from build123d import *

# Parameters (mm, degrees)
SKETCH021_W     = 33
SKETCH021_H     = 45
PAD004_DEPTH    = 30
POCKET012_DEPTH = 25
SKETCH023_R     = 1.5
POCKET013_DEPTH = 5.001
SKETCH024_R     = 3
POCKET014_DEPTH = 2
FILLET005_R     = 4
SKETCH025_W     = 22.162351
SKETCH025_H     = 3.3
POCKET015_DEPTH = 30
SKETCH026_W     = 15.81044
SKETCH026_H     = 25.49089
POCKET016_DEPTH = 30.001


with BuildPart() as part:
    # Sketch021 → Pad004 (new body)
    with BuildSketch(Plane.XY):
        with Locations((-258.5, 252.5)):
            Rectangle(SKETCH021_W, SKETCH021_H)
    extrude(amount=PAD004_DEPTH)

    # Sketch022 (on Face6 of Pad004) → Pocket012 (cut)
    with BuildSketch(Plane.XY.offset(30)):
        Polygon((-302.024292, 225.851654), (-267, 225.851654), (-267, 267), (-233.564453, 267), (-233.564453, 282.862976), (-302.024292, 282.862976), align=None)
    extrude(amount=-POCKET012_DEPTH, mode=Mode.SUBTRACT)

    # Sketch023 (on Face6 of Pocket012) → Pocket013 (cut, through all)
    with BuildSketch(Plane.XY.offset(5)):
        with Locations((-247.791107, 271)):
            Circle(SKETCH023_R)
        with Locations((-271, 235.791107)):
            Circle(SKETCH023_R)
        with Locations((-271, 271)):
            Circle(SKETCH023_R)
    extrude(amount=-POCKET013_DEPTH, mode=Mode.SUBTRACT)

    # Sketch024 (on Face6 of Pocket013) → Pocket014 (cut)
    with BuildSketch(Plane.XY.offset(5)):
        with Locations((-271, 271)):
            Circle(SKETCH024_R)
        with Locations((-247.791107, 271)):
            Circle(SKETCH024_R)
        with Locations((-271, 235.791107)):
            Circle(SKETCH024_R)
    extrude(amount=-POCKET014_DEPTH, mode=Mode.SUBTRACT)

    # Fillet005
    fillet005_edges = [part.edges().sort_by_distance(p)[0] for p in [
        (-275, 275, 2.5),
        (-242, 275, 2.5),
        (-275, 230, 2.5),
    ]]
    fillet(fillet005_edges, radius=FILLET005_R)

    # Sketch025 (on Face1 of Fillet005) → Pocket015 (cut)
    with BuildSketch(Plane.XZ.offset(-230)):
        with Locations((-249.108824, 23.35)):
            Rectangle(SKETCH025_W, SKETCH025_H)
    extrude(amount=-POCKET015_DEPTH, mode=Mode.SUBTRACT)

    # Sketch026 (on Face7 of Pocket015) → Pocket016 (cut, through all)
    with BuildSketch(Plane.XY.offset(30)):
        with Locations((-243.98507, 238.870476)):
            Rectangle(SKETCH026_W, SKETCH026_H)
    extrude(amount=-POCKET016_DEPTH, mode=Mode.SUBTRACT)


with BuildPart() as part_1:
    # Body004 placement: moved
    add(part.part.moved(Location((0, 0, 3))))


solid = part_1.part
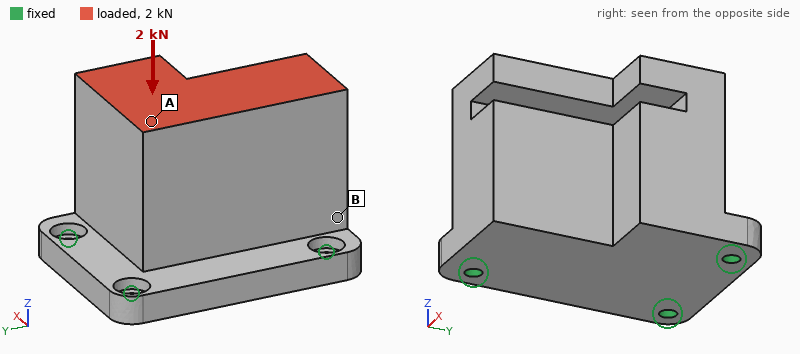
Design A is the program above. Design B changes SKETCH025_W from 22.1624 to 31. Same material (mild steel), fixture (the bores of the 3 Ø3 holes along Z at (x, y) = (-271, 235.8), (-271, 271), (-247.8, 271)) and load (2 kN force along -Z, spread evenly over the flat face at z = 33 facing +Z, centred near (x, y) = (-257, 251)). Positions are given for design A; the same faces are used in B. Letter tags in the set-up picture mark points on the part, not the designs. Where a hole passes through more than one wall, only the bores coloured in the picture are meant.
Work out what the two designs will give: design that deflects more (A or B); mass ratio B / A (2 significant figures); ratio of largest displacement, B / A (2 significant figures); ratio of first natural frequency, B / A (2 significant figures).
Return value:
B
0.98
1.9
1.0
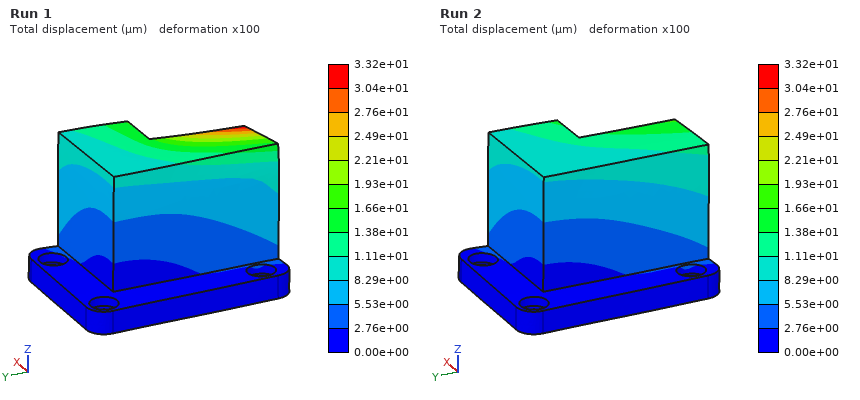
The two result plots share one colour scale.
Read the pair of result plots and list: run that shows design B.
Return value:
Run 1
